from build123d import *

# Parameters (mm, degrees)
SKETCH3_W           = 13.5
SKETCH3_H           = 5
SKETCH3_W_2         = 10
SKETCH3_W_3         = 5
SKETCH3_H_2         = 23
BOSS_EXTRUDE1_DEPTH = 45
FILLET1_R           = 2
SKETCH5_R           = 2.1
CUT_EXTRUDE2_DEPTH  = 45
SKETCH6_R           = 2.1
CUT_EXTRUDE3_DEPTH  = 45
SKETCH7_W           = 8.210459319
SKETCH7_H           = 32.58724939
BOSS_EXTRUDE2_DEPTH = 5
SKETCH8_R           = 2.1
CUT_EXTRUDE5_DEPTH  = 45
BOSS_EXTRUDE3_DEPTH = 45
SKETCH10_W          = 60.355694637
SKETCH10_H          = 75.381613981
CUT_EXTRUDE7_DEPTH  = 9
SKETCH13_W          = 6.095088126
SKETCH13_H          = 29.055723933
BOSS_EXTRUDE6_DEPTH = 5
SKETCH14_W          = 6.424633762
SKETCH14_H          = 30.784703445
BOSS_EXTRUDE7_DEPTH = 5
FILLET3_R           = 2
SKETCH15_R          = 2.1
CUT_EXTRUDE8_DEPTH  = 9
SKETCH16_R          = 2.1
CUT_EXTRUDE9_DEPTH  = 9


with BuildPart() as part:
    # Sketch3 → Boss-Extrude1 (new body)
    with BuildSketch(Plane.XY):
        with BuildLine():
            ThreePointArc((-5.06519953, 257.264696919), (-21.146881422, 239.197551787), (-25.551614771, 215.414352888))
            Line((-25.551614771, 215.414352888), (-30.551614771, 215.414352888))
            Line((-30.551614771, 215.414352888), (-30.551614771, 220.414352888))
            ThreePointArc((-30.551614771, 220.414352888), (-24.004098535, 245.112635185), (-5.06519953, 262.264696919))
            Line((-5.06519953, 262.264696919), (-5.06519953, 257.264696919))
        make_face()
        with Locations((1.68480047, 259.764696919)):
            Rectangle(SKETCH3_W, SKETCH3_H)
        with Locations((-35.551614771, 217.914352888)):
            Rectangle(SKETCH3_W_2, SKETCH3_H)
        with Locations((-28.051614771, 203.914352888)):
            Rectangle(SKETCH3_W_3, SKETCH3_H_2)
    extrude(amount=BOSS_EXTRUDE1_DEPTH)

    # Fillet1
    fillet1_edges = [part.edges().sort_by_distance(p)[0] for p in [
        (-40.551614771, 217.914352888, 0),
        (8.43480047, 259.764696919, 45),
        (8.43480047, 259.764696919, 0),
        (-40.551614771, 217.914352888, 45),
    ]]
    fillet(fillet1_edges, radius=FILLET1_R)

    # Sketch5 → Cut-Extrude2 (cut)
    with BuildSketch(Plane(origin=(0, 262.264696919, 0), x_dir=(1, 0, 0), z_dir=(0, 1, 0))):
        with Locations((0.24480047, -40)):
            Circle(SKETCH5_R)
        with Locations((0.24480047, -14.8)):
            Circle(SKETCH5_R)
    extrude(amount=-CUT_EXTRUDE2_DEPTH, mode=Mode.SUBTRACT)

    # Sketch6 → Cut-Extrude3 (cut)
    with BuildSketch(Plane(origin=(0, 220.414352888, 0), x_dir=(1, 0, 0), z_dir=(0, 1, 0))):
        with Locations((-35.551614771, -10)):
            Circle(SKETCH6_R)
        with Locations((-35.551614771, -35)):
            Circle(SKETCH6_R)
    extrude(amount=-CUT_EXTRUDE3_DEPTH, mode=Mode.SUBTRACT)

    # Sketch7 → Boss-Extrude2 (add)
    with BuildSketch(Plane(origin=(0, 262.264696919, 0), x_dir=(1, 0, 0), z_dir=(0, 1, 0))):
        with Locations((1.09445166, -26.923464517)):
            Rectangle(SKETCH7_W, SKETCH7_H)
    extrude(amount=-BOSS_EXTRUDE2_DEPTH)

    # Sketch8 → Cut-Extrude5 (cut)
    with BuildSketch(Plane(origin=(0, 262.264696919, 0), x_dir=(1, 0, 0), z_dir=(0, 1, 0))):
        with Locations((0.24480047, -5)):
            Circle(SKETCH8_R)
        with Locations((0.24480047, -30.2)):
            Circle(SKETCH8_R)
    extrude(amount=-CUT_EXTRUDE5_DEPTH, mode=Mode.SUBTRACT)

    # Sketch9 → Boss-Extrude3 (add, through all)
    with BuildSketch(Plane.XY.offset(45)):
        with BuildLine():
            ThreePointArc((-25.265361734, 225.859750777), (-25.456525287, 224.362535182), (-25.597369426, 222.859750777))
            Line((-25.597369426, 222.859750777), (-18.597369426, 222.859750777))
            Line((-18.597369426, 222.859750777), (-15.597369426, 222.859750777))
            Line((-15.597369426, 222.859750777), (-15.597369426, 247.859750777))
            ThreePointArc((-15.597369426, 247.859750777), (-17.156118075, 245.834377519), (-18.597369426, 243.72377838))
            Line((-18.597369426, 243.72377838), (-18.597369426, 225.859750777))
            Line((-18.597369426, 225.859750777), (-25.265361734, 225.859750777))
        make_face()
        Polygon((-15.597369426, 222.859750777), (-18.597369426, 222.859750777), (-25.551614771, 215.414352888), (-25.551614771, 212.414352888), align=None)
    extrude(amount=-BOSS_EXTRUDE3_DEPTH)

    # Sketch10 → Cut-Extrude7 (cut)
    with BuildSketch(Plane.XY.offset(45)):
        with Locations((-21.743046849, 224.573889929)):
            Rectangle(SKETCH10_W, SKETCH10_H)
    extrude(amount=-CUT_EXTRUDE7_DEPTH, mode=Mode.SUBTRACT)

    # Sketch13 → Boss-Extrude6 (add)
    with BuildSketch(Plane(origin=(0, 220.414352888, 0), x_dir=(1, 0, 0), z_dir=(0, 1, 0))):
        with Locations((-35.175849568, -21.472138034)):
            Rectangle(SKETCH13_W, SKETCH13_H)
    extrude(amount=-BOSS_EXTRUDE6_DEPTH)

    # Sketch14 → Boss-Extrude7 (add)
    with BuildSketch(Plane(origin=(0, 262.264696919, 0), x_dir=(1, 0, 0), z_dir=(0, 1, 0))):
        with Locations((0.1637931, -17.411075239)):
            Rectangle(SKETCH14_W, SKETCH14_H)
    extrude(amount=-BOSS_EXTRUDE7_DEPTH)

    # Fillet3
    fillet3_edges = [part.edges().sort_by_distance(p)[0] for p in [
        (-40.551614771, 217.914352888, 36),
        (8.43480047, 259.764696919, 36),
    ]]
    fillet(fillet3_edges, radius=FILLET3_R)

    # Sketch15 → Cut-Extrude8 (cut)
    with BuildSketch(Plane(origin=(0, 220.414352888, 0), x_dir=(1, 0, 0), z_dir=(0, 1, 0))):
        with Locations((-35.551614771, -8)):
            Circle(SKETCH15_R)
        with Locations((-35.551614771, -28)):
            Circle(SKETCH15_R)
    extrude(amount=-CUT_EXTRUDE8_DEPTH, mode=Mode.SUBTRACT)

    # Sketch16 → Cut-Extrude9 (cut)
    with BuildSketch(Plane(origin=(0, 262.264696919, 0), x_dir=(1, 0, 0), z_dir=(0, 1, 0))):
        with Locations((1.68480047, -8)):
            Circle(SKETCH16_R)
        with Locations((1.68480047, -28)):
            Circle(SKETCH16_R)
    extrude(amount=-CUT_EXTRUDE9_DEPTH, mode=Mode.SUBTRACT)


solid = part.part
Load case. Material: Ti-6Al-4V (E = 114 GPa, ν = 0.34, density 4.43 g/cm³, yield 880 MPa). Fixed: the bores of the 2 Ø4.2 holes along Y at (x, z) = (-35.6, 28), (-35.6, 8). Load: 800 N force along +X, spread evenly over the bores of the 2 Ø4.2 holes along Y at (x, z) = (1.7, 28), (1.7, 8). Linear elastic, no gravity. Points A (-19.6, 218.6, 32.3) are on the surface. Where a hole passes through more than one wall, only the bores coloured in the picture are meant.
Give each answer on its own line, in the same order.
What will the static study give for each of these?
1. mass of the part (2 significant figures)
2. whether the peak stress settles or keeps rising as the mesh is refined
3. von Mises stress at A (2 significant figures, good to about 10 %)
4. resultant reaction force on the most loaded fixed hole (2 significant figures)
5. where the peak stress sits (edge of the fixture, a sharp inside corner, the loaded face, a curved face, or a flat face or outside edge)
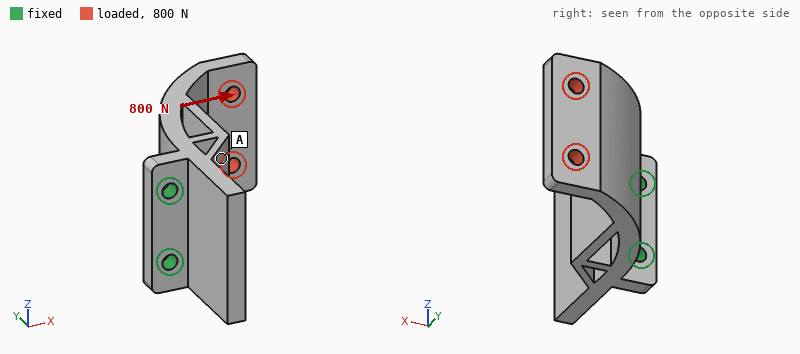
97 g
keeps rising
31 MPa
430 N
edge of the fixture
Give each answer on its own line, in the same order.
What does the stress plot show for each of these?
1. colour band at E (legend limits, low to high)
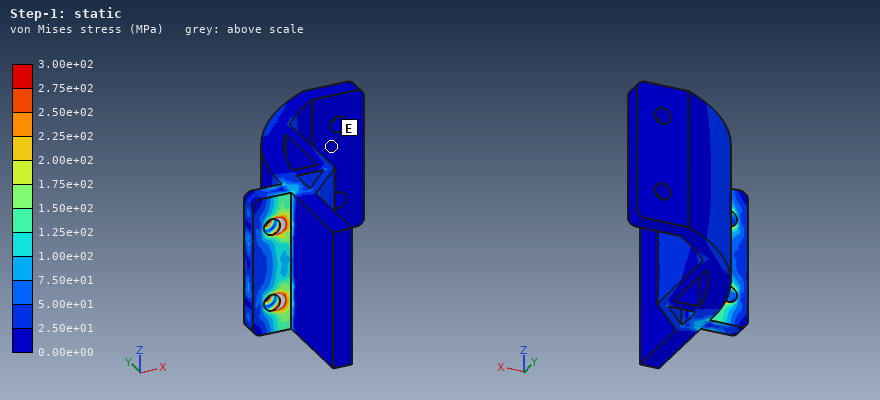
0.00e+00 to 2.50e+01 MPa
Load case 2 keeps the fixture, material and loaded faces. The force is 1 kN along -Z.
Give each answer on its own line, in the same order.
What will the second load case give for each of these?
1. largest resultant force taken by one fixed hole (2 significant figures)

2.5 kN
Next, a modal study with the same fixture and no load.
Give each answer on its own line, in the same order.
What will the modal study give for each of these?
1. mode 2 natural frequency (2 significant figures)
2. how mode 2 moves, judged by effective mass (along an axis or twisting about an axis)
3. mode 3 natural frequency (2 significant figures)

3900 Hz
along Z
5100 Hz
